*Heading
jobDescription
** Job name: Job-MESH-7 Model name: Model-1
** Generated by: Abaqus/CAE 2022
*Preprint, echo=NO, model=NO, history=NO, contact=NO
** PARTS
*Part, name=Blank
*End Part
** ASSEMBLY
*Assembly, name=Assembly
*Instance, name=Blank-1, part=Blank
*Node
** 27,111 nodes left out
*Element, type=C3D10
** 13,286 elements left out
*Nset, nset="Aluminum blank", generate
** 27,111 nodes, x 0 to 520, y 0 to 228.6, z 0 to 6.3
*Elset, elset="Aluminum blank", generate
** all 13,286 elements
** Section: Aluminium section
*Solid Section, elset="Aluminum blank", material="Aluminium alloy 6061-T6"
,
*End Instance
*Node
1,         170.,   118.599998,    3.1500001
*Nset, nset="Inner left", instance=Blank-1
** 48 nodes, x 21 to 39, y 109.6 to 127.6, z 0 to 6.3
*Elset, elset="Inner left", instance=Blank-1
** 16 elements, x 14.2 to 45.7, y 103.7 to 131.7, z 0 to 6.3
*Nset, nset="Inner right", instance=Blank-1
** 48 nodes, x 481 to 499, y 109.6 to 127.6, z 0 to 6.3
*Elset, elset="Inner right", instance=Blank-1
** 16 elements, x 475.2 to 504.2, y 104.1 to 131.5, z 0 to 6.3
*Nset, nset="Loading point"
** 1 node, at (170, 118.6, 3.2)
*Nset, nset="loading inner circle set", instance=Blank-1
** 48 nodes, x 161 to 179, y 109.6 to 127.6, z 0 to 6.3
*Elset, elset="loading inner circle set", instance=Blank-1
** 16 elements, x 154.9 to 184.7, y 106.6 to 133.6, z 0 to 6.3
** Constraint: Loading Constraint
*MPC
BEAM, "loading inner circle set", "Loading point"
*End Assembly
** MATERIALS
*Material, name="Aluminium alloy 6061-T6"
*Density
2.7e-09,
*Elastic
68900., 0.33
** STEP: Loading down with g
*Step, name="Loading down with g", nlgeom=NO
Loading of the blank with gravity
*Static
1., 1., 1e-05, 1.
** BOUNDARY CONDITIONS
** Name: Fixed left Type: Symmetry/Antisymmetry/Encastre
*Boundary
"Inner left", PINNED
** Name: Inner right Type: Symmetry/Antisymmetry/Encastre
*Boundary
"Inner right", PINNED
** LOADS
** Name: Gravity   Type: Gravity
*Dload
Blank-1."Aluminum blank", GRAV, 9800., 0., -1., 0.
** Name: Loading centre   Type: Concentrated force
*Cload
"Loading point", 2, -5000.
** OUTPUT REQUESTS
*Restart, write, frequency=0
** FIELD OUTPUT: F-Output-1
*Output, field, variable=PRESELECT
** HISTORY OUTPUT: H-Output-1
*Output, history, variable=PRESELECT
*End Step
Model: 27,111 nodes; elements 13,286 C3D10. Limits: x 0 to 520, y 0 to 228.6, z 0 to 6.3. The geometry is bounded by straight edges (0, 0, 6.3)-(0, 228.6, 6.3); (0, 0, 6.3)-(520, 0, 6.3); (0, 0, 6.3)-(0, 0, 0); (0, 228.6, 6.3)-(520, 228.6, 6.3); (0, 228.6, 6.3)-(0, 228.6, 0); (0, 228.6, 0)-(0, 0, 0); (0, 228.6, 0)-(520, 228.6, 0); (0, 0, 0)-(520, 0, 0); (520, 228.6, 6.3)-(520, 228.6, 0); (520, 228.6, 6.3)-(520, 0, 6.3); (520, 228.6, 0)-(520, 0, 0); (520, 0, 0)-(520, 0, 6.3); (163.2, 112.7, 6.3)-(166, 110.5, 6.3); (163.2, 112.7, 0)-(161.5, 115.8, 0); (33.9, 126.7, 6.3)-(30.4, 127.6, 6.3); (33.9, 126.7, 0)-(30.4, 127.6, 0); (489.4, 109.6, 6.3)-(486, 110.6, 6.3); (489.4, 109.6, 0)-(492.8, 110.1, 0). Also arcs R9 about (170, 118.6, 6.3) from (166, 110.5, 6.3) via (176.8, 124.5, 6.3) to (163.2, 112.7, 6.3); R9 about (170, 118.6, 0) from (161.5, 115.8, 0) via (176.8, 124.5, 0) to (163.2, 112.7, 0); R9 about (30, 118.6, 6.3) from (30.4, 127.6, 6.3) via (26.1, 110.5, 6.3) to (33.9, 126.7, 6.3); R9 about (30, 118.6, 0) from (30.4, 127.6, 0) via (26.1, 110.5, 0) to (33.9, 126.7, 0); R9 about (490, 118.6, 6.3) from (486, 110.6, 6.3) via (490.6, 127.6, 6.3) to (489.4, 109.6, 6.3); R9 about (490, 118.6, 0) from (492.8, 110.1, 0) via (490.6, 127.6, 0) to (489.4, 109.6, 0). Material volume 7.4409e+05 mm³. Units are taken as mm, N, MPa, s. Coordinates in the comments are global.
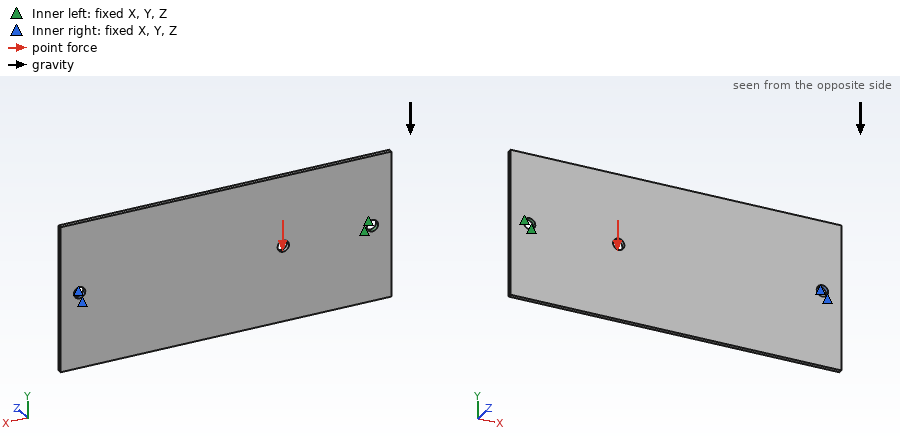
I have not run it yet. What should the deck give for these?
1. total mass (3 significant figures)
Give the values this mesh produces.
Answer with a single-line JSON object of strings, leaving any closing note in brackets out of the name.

{"total mass": "2.01 kg"}
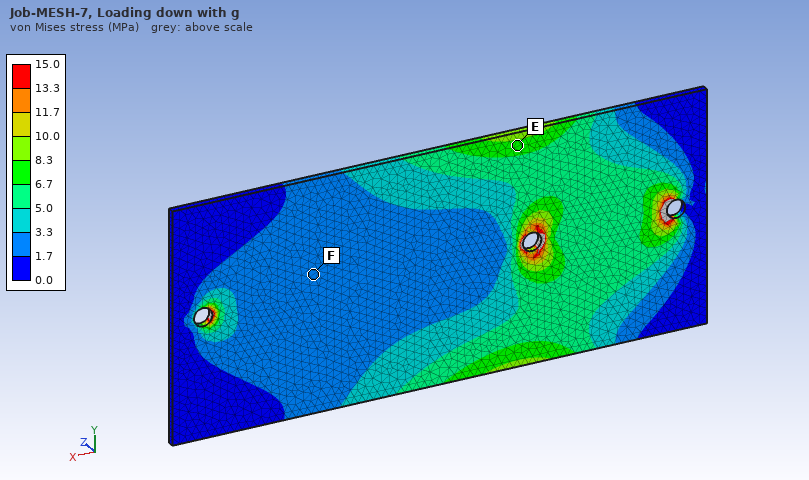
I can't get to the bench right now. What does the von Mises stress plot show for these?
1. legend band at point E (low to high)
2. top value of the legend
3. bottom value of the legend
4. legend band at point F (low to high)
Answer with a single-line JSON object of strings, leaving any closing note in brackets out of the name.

{"legend band at point E": "6.7 to 8.3 MPa", "top value of the legend": "15.0 MPa", "bottom value of the legend": "0.0 MPa", "legend band at point F": "1.7 to 3.3 MPa"}
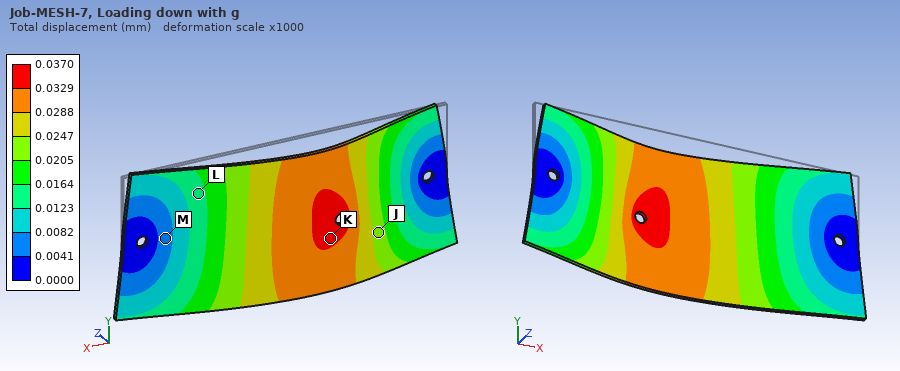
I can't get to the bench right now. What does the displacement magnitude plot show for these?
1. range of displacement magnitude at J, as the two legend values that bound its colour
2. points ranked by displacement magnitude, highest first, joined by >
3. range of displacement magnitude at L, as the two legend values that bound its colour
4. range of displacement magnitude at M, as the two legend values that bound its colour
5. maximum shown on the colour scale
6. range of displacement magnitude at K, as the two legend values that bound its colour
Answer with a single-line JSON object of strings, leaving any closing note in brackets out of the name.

{"range of displacement magnitude at J, as the two legend values that bound its colour": "0.0205 to 0.0247 mm", "points ranked by displacement magnitude, highest first, joined by >": "K > J > L > M", "range of displacement magnitude at L, as the two legend values that bound its colour": "0.0123 to 0.0164 mm", "range of displacement magnitude at M, as the two legend values that bound its colour": "0.0041 to 0.0082 mm", "maximum shown on the colour scale": "0.0370 mm", "range of displacement magnitude at K, as the two legend values that bound its colour": "0.0329 to 0.0370 mm"}
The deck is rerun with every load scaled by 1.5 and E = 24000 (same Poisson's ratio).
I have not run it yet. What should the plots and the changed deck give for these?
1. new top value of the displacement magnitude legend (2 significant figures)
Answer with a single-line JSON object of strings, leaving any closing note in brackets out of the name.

{"new top value of the displacement magnitude legend": "0.16 mm"}
